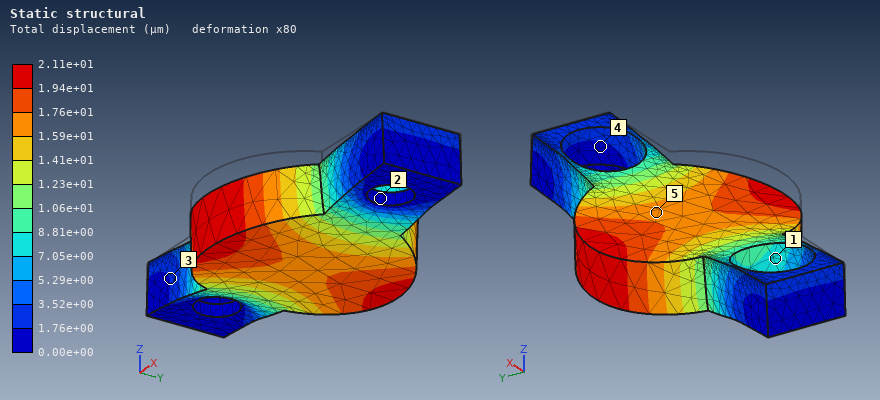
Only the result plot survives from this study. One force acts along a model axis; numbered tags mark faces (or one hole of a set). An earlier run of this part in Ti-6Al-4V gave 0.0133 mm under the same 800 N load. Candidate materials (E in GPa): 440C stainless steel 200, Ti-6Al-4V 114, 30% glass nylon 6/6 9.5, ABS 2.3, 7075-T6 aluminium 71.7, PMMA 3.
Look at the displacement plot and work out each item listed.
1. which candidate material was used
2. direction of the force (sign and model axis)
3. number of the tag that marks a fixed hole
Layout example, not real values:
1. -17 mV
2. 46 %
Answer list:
1. 7075-T6 aluminium
2. -Z
3. 2
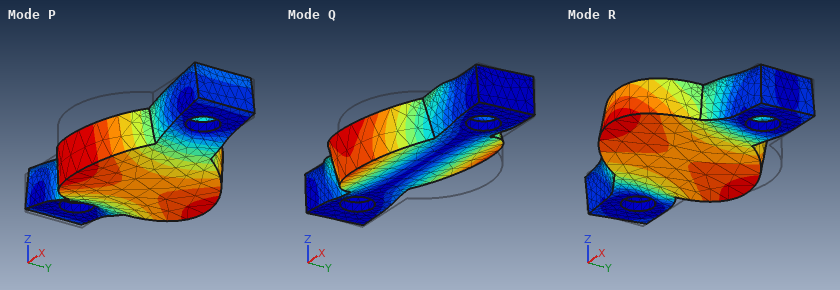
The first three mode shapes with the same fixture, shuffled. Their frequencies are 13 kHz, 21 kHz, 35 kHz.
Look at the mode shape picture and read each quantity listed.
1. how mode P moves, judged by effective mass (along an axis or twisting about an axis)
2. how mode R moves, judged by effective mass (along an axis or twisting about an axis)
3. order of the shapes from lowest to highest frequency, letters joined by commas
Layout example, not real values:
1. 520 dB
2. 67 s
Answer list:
1. along Z
2. along Y
3. Q, P, R
